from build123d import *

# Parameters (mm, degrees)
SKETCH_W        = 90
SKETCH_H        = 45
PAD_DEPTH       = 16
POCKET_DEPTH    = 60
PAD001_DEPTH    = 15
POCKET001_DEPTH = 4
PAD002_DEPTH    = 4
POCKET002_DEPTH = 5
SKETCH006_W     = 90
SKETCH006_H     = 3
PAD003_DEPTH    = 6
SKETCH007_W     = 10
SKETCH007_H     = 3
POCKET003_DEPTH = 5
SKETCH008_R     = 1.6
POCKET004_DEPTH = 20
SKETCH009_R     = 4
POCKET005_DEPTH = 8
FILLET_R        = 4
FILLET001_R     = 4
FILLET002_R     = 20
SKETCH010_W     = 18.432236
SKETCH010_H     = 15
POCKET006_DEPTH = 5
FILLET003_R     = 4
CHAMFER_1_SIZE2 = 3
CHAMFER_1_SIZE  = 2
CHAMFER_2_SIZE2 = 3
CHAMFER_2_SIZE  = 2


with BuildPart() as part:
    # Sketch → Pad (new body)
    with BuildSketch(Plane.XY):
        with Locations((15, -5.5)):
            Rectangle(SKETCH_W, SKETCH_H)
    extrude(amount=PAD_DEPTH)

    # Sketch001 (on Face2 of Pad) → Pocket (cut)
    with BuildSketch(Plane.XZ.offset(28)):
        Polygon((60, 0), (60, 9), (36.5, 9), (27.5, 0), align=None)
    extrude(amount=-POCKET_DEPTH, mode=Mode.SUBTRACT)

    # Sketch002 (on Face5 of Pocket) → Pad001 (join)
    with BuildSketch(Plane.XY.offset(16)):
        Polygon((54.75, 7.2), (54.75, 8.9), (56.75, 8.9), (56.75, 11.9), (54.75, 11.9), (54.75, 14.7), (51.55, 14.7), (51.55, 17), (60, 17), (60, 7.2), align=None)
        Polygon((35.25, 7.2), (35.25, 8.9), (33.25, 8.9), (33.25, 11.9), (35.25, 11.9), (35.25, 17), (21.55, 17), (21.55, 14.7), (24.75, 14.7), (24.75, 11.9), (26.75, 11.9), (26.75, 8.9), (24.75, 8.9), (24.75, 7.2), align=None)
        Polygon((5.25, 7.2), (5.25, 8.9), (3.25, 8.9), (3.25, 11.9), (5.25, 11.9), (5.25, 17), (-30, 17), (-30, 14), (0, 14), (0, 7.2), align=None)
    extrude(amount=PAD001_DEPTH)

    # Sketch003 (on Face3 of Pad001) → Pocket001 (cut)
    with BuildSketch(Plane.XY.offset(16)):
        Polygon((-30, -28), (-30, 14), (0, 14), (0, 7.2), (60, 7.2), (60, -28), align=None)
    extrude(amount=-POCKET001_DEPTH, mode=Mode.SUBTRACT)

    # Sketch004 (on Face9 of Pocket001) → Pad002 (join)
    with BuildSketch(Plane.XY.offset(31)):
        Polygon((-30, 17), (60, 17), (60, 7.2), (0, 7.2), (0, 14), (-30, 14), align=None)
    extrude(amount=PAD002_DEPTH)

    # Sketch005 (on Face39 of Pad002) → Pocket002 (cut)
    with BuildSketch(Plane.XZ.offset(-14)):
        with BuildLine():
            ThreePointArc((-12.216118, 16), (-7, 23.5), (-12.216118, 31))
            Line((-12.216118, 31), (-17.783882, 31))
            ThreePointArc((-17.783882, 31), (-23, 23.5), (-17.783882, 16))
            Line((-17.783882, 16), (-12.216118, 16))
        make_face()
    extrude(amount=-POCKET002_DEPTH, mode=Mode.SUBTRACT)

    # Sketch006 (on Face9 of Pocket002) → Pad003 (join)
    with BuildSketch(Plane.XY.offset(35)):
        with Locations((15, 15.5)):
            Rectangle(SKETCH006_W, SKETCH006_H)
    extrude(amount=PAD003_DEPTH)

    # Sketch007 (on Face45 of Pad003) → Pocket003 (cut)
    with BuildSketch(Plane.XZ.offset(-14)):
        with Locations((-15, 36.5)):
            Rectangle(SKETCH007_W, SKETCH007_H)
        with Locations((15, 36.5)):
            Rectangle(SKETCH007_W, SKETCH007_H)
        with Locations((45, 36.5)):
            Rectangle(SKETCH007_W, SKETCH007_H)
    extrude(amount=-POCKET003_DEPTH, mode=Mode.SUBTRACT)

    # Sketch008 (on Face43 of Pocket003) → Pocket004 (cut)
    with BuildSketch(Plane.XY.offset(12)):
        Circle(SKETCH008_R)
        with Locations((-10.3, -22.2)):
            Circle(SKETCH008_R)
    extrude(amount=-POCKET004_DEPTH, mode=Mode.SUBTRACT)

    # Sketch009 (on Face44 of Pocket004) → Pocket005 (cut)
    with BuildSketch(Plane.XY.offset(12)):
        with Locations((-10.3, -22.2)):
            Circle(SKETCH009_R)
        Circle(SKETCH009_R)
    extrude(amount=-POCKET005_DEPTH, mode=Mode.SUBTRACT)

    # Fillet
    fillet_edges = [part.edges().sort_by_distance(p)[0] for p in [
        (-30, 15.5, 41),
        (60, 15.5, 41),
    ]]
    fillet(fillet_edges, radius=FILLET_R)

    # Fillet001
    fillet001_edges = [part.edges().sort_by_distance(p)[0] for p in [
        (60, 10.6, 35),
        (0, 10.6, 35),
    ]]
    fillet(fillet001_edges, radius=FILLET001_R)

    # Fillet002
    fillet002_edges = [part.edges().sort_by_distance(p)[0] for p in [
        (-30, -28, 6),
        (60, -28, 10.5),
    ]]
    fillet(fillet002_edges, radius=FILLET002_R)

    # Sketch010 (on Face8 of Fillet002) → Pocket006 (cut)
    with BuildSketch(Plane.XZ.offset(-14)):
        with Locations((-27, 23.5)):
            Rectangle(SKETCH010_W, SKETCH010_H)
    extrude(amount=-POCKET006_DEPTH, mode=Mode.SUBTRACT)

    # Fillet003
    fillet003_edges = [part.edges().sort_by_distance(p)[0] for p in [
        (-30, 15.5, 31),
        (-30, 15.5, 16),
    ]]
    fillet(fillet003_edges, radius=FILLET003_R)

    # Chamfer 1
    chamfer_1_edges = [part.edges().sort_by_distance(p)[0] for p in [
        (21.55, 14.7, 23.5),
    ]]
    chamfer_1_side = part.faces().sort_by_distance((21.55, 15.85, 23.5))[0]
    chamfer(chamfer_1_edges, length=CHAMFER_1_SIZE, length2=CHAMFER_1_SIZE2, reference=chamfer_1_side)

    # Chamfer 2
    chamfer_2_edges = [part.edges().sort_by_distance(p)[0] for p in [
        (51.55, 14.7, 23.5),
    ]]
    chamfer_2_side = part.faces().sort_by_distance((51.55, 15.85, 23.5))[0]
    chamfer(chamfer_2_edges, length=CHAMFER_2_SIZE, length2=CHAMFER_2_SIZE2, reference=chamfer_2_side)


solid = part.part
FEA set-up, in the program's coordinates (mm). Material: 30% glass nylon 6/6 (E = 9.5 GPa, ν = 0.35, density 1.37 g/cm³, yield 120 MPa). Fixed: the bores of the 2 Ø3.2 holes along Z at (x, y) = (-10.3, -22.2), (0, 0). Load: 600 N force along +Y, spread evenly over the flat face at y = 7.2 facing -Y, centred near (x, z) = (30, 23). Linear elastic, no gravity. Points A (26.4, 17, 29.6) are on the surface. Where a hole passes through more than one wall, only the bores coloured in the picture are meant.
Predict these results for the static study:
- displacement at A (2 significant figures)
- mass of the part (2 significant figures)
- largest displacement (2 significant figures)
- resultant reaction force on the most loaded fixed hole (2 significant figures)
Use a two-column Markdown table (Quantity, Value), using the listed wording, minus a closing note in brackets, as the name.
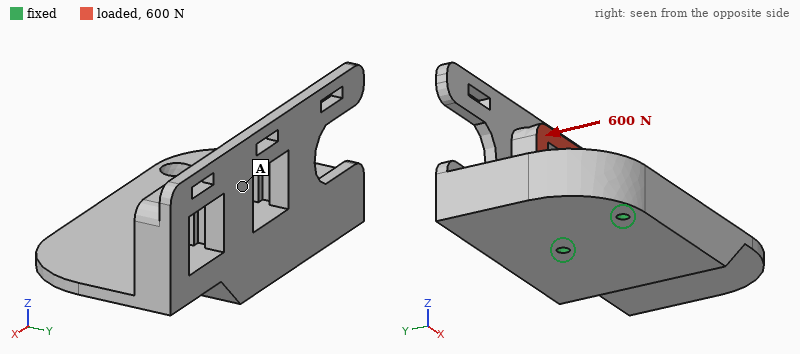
| Quantity | Value |
|---|---|
| displacement at A | 0.39 mm |
| mass of the part | 62 g |
| largest displacement | 0.73 mm |
| resultant reaction force on the most loaded fixed hole | 1.0 kN |
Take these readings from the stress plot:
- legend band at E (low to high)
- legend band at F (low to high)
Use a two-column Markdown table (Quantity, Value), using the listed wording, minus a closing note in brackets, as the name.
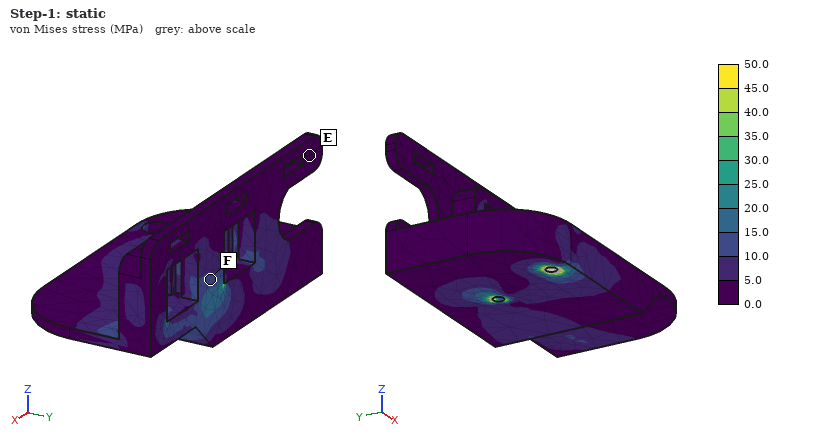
| Quantity | Value |
|---|---|
| legend band at E | 0.0 to 5.0 MPa |
| legend band at F | 10.0 to 15.0 MPa |
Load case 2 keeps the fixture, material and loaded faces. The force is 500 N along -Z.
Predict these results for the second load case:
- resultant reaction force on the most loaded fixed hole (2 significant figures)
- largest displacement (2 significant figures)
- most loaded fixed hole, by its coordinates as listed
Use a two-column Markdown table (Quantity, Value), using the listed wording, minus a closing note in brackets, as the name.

| Quantity | Value |
|---|---|
| resultant reaction force on the most loaded fixed hole | 860 N |
| largest displacement | 1.3 mm |
| most loaded fixed hole, by its coordinates as listed | (0, 0) |
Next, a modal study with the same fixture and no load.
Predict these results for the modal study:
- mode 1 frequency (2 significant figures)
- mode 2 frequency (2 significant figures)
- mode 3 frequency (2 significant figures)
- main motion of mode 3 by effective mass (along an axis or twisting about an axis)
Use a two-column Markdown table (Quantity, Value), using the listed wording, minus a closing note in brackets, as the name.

| Quantity | Value |
|---|---|
| mode 1 frequency | 640 Hz |
| mode 2 frequency | 1400 Hz |
| mode 3 frequency | 1600 Hz |
| main motion of mode 3 by effective mass | along Y |
